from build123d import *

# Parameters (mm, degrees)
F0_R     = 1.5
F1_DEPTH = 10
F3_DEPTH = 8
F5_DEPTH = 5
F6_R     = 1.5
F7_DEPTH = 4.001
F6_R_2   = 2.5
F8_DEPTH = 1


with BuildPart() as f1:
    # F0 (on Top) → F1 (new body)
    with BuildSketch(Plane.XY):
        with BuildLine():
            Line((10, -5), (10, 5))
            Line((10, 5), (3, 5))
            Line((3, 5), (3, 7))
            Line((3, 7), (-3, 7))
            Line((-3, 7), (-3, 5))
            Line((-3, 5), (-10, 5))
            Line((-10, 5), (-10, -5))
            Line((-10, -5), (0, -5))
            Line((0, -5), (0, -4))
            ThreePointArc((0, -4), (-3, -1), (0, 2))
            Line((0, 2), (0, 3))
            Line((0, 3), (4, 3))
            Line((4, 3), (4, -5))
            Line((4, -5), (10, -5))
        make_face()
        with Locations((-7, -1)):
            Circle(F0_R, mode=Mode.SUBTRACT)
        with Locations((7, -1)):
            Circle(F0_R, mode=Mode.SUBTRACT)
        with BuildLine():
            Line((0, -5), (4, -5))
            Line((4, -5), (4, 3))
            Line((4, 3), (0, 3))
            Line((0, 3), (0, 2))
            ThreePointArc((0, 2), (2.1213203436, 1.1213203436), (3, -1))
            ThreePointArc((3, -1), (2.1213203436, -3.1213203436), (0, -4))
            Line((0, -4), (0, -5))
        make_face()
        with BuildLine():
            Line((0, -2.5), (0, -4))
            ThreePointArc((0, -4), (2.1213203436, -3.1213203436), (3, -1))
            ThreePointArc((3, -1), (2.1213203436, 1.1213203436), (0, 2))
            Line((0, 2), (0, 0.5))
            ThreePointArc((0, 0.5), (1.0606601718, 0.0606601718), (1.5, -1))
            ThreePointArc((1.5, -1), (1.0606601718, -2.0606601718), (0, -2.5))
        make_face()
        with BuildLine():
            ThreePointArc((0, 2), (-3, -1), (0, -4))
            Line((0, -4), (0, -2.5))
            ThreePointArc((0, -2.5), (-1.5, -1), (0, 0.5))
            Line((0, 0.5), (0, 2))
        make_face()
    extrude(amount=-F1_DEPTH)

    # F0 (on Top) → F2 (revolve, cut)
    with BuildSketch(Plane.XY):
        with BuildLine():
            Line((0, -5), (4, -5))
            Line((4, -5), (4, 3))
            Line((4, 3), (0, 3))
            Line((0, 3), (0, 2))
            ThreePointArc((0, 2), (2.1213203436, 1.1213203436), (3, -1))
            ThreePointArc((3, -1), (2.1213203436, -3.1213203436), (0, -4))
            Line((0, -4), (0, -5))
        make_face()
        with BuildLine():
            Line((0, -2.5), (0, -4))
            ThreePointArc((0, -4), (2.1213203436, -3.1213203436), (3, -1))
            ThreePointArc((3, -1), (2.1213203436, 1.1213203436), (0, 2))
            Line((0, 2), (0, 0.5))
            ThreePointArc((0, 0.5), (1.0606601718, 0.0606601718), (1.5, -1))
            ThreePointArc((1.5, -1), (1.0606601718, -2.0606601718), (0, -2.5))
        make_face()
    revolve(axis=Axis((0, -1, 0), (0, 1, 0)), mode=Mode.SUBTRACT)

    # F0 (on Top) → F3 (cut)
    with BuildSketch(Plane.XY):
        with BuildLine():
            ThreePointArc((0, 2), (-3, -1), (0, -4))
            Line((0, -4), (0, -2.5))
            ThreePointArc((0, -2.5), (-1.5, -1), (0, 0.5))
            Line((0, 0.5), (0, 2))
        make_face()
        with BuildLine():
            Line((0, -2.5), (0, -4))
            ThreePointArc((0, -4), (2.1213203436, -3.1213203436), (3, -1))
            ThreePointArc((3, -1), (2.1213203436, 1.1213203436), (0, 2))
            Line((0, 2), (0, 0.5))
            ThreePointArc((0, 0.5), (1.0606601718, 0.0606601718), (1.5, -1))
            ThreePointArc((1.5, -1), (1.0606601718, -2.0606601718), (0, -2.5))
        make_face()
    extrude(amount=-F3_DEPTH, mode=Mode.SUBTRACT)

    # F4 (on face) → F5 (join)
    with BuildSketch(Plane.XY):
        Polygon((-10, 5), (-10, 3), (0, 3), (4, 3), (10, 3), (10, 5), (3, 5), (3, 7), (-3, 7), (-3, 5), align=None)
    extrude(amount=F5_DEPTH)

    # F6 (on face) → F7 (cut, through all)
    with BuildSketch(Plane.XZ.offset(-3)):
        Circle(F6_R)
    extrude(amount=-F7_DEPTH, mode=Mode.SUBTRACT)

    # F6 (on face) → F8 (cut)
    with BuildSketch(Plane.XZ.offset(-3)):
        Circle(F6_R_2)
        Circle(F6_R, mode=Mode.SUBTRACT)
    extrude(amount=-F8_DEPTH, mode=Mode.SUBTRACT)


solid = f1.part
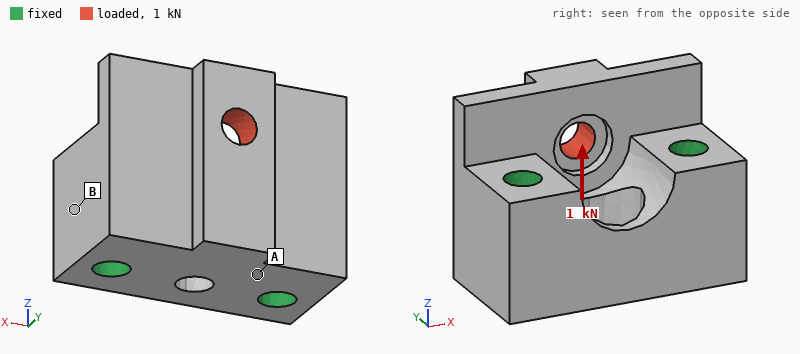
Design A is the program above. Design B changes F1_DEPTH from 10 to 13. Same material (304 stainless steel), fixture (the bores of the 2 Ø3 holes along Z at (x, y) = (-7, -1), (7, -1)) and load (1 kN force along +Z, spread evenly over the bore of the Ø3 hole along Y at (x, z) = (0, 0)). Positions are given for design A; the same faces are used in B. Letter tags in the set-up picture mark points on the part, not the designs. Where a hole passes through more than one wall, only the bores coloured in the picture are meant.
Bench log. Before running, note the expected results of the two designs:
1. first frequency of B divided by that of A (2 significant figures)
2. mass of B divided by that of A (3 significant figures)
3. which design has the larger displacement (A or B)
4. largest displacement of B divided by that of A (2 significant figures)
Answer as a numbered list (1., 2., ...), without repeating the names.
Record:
1. 1.0
2. 1.31
3. A
4. 0.86
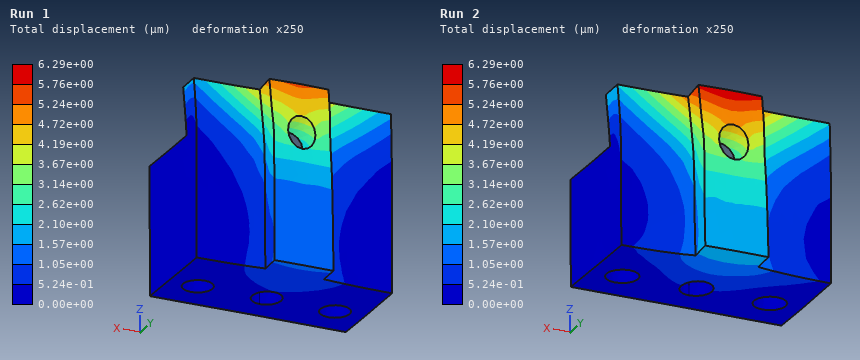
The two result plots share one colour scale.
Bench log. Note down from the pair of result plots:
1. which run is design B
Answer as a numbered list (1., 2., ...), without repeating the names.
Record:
1. Run 1
